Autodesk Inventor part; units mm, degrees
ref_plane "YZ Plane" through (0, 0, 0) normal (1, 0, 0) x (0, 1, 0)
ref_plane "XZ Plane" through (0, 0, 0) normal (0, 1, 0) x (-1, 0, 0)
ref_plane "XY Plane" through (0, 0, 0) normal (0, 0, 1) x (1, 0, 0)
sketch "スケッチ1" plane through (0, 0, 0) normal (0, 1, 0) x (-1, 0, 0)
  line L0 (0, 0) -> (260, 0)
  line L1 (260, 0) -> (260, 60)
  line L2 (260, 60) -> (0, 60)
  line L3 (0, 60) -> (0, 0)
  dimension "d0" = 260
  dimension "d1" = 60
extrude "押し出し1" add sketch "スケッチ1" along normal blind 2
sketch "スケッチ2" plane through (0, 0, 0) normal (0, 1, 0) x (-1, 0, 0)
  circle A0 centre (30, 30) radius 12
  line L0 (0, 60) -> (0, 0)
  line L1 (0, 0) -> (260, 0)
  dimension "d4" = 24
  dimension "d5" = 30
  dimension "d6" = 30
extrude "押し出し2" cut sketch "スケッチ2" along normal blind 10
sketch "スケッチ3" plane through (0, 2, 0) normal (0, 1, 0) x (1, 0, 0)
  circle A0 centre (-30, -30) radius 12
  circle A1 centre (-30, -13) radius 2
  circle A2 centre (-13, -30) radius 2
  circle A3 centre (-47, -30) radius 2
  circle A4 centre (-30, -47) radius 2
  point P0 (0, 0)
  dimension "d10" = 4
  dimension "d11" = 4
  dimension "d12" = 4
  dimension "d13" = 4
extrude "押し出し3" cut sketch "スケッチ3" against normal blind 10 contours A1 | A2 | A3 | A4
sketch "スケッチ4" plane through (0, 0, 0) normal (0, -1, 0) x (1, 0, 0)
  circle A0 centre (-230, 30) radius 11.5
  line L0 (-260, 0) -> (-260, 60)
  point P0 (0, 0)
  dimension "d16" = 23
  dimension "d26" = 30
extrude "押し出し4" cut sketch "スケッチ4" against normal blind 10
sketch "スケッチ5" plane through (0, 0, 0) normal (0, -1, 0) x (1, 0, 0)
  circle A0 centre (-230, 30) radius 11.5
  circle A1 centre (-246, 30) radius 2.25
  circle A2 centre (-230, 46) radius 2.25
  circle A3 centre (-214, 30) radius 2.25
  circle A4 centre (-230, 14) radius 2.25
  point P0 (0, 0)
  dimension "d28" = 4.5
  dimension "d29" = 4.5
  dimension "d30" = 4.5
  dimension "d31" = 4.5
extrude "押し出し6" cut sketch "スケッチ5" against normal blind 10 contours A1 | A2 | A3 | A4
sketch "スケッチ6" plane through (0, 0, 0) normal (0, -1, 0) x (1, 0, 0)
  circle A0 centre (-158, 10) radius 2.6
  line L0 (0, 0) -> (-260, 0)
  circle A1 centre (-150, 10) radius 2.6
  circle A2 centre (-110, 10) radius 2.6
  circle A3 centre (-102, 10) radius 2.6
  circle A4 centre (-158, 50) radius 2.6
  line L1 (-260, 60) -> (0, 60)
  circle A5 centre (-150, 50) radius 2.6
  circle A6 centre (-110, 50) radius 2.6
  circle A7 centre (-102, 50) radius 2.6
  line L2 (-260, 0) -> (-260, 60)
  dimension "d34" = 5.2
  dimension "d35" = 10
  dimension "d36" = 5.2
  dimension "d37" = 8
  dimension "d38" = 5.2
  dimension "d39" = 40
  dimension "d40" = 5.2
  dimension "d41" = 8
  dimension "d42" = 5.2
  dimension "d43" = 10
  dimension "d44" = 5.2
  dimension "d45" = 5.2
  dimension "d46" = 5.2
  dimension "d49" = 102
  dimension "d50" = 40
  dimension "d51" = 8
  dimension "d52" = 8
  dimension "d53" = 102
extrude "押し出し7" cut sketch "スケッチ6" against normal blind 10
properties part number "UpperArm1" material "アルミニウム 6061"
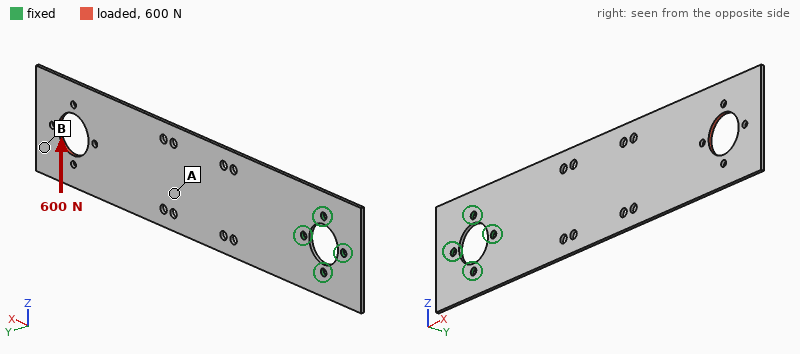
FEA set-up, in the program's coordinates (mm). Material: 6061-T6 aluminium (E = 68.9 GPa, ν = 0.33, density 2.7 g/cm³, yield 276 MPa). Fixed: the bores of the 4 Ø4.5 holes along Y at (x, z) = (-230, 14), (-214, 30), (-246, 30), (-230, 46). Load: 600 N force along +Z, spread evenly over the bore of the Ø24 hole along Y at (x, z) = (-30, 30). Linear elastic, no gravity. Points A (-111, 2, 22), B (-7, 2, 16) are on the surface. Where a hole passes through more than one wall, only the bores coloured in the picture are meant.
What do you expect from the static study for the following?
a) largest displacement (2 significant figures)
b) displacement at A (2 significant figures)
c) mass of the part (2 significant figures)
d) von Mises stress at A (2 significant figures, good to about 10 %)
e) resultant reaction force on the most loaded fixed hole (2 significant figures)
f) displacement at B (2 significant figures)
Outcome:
0.95 mm
0.34 mm
78 g
18 MPa
2.5 kN
0.91 mm
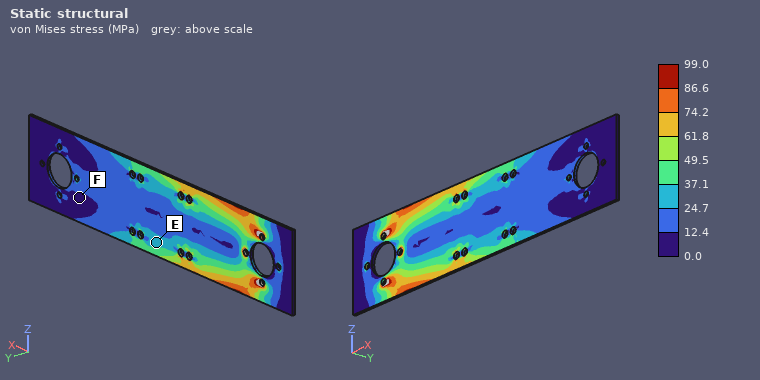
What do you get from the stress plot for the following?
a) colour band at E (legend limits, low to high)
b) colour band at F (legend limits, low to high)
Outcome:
24.7 to 37.1 MPa
0.0 to 12.4 MPa
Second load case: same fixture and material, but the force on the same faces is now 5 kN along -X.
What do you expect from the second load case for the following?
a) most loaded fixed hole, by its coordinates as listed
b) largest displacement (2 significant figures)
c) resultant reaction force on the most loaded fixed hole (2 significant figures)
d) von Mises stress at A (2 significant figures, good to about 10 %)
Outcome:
(-214, 30)
0.16 mm
2.2 kN
44 MPa
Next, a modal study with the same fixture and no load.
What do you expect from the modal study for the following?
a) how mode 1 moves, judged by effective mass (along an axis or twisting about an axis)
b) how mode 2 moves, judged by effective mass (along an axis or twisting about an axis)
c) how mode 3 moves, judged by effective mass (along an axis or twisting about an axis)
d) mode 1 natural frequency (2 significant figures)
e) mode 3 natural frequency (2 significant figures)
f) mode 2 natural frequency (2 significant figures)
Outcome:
along Y
along Y
twisting about X
37 Hz
240 Hz
220 Hz
